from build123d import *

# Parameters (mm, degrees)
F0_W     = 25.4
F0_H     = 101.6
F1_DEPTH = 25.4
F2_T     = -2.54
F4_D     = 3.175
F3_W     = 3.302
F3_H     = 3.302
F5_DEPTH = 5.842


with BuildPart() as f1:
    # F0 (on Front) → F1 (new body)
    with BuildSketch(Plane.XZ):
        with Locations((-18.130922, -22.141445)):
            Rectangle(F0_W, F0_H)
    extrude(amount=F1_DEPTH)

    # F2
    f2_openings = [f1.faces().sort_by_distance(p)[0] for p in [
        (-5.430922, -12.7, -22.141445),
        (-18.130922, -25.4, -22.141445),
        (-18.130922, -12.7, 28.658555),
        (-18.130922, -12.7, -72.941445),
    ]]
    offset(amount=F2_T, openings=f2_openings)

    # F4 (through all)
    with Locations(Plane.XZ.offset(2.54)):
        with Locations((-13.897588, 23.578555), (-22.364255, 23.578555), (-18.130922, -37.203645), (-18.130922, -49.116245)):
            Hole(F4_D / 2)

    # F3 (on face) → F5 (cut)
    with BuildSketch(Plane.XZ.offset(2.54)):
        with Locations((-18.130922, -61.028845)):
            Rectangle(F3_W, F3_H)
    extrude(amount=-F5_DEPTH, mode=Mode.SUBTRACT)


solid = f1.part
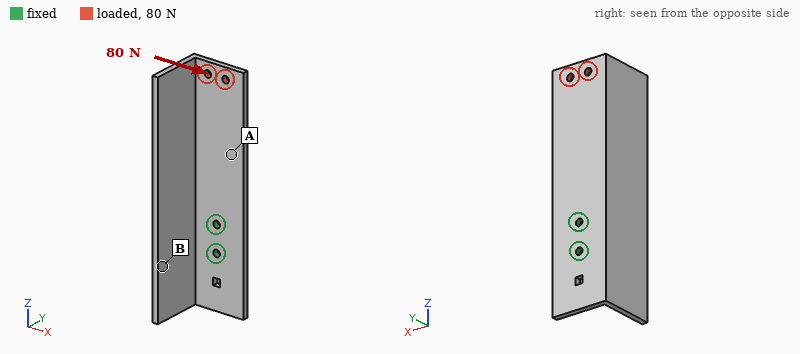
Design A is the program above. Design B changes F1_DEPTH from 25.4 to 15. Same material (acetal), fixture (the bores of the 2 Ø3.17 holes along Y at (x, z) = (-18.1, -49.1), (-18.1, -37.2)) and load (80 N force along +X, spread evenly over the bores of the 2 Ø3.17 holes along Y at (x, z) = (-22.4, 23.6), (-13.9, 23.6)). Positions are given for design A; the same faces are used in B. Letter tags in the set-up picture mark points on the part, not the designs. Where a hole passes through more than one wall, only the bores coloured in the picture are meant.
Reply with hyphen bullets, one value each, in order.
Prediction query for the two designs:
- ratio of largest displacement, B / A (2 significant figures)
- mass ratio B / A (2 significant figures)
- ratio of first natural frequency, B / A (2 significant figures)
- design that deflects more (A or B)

- 1.2
- 0.78
- 1.1
- B
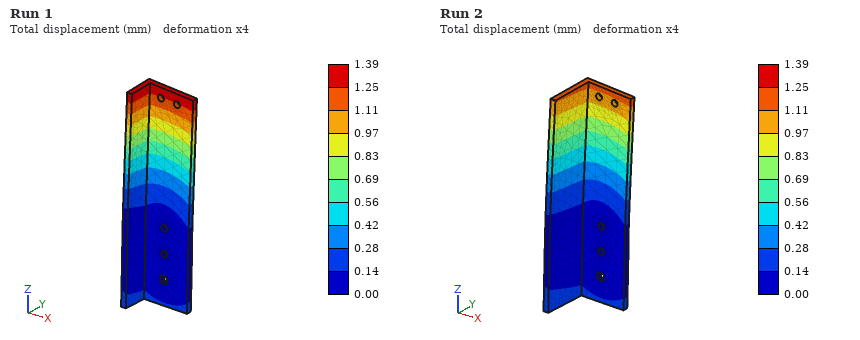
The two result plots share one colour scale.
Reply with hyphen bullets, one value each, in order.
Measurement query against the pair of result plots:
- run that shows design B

- Run 1
